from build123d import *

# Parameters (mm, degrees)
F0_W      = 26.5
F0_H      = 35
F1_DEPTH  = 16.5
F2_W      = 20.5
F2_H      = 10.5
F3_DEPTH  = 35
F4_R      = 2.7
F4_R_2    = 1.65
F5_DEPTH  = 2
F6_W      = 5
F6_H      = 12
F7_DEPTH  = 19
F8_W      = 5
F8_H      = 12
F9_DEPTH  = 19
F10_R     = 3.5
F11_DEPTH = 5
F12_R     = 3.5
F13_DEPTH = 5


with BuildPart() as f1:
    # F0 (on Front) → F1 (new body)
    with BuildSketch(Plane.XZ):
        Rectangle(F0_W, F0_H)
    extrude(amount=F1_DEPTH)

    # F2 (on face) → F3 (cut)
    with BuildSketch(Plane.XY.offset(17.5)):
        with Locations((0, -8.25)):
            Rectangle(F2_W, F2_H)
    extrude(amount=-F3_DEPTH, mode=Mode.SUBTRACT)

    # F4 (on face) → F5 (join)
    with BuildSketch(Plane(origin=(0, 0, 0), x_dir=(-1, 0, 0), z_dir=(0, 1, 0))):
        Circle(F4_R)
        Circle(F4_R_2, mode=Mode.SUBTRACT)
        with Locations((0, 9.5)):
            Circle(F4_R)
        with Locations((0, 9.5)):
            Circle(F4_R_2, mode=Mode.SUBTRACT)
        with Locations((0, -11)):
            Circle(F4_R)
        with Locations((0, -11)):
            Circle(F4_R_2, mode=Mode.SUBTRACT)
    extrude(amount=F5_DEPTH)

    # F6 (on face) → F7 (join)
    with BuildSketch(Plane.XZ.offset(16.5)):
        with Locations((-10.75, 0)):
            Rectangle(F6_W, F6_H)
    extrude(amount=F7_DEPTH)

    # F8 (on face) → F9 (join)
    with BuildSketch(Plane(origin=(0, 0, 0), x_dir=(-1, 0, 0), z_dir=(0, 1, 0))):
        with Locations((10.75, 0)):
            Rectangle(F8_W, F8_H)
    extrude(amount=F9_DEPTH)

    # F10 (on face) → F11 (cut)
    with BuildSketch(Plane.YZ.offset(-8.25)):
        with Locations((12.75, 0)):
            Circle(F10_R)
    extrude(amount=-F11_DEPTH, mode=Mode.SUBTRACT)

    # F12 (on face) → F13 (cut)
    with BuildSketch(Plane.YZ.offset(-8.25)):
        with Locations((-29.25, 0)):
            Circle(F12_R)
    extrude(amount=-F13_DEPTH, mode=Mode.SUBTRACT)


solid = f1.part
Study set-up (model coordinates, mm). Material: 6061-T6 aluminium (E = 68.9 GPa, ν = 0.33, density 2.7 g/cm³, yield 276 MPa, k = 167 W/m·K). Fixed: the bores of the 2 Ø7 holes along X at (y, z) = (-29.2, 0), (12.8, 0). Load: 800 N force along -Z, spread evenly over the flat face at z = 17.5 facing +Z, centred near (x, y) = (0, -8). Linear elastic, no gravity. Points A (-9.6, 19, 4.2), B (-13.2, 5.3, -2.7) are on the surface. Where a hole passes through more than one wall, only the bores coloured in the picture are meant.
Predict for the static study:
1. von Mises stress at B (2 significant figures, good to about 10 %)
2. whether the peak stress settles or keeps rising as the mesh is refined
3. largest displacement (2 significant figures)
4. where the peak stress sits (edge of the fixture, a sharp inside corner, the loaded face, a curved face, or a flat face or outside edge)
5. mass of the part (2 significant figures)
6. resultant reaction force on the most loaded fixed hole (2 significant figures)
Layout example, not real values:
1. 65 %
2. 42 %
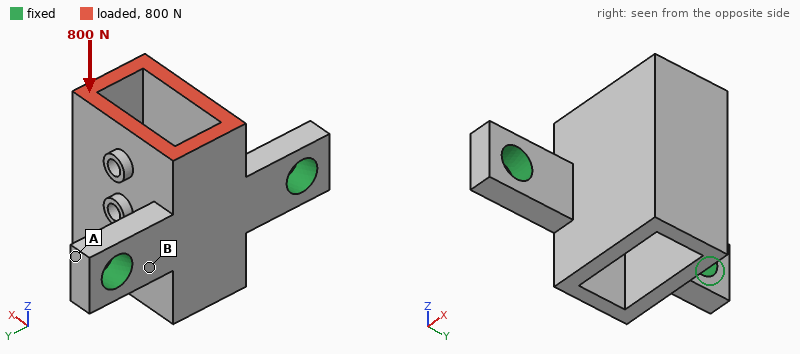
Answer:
1. 58 MPa
2. keeps rising
3. 0.14 mm
4. edge of the fixture
5. 26 g
6. 400 N
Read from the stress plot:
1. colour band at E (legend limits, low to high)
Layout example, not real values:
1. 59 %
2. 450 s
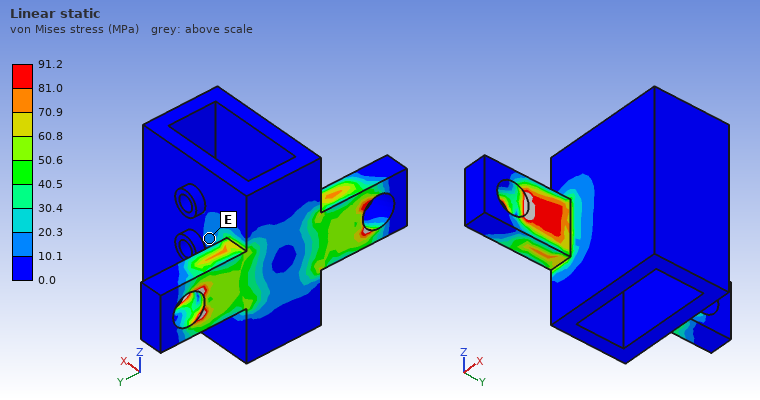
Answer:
1. 10.1 to 20.3 MPa
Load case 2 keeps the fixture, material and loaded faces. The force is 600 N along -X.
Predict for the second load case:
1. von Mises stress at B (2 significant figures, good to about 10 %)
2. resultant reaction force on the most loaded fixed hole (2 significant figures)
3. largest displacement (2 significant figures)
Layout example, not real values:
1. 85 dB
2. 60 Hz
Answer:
1. 86 MPa
2. 310 N
3. 0.17 mm
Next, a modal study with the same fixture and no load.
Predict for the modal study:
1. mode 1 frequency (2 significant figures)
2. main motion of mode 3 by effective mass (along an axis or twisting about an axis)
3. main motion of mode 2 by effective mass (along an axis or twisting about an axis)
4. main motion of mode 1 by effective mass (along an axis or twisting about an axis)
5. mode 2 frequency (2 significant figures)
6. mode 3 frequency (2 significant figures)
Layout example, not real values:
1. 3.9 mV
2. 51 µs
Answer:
1. 2800 Hz
2. along X
3. along Y
4. along Z
5. 4800 Hz
6. 7600 Hz
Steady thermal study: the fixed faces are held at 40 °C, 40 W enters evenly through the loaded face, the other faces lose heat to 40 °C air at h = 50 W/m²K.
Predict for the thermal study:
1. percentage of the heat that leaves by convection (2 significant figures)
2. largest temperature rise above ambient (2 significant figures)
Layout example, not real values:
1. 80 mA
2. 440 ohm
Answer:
1. 19 %
2. 44 K
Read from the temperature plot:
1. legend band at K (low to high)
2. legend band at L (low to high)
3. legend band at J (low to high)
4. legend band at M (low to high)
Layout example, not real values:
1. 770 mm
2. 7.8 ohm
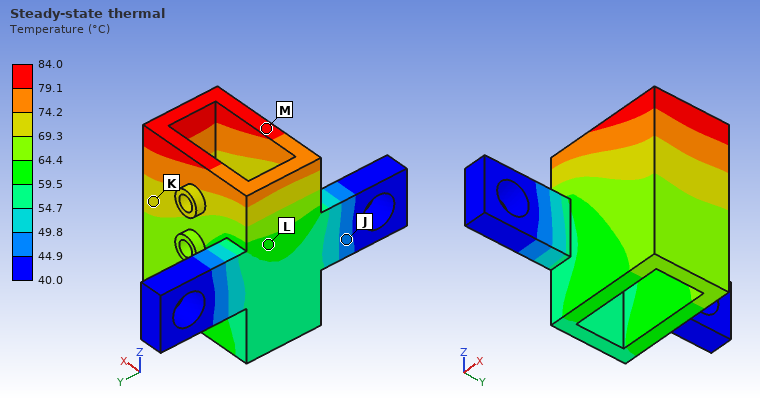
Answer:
1. 69.3 to 74.2 °C
2. 59.5 to 64.4 °C
3. 44.9 to 49.8 °C
4. 79.1 to 84.0 °C
